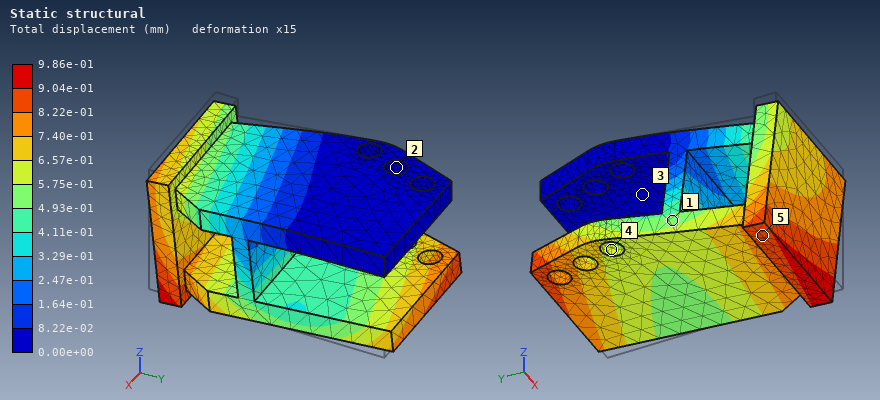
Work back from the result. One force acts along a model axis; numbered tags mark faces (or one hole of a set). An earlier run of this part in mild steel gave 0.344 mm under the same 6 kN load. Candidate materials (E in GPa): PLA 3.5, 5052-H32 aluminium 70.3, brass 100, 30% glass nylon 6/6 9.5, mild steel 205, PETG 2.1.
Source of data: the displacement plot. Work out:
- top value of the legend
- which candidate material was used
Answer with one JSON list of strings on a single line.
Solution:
["9.86e-01 mm", "5052-H32 aluminium"]
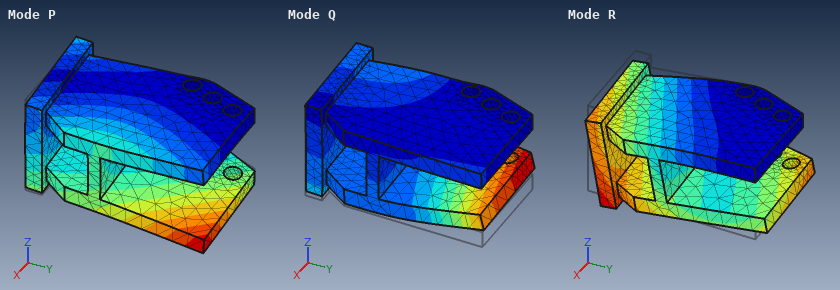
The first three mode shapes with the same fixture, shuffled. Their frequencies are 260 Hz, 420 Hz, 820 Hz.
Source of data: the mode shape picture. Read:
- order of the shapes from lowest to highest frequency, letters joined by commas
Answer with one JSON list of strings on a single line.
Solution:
["R, P, Q"]
